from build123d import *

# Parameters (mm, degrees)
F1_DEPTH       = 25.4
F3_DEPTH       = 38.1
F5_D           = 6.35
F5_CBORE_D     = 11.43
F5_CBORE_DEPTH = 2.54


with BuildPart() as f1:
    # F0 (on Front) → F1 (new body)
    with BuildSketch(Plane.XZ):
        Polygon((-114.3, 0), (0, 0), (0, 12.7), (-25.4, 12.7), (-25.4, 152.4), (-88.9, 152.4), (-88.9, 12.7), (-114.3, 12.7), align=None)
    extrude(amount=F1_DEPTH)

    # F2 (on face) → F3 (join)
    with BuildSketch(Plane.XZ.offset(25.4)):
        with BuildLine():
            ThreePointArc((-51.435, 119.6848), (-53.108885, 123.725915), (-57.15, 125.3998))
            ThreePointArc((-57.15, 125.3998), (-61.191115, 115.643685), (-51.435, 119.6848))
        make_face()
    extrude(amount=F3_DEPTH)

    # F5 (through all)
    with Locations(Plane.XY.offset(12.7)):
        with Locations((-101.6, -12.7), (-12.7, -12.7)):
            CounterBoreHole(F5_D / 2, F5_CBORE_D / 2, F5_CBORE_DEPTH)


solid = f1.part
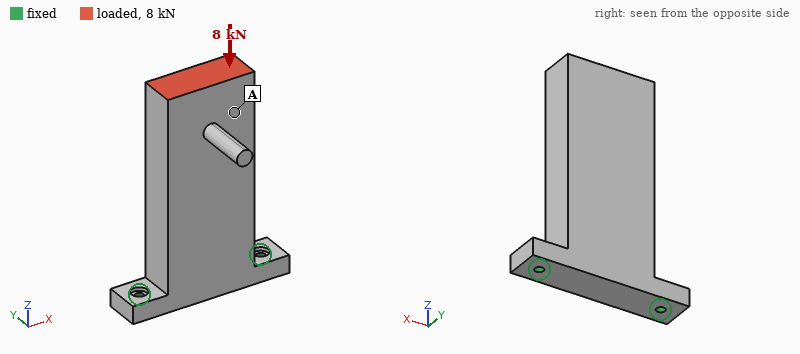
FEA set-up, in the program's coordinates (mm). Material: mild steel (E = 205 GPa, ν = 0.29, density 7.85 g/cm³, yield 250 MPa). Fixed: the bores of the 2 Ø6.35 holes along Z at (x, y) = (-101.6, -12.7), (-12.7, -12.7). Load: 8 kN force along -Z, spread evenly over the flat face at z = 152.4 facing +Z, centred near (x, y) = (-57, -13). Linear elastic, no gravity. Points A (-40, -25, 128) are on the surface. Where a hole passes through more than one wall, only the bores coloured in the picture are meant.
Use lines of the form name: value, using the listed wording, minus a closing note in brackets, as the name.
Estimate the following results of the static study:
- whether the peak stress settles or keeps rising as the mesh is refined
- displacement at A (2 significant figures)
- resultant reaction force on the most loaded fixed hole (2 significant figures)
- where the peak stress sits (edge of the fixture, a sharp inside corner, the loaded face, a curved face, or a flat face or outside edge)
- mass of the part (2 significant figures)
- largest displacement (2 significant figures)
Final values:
whether the peak stress settles or keeps rising as the mesh is refined: keeps rising
displacement at A: 9.9 µm
resultant reaction force on the most loaded fixed hole: 4.6 kN
where the peak stress sits: edge of the fixture
mass of the part: 2.1 kg
largest displacement: 11 µm
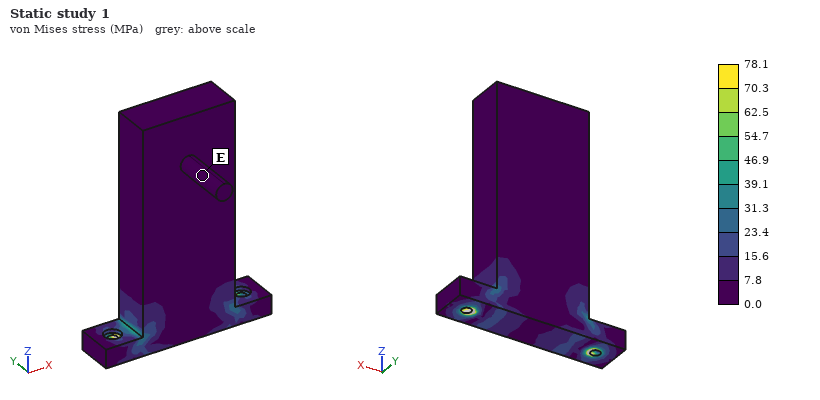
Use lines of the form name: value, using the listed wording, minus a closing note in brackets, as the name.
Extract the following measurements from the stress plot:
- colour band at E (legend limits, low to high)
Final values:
colour band at E: 0.0 to 7.8 MPa
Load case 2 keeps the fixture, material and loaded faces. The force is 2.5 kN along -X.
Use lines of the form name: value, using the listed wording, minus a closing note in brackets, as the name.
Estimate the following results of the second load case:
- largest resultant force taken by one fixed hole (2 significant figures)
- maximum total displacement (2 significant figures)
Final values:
largest resultant force taken by one fixed hole: 5.0 kN
maximum total displacement: 56 µm
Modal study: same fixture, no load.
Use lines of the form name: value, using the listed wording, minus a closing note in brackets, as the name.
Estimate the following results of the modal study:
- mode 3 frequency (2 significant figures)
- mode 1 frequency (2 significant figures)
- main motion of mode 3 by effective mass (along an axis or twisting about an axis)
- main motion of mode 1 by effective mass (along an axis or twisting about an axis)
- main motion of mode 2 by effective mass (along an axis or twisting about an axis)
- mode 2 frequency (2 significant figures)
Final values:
mode 3 frequency: 3200 Hz
mode 1 frequency: 390 Hz
main motion of mode 3 by effective mass: twisting about Z
main motion of mode 1 by effective mass: along Y
main motion of mode 2 by effective mass: along X
mode 2 frequency: 1400 Hz
